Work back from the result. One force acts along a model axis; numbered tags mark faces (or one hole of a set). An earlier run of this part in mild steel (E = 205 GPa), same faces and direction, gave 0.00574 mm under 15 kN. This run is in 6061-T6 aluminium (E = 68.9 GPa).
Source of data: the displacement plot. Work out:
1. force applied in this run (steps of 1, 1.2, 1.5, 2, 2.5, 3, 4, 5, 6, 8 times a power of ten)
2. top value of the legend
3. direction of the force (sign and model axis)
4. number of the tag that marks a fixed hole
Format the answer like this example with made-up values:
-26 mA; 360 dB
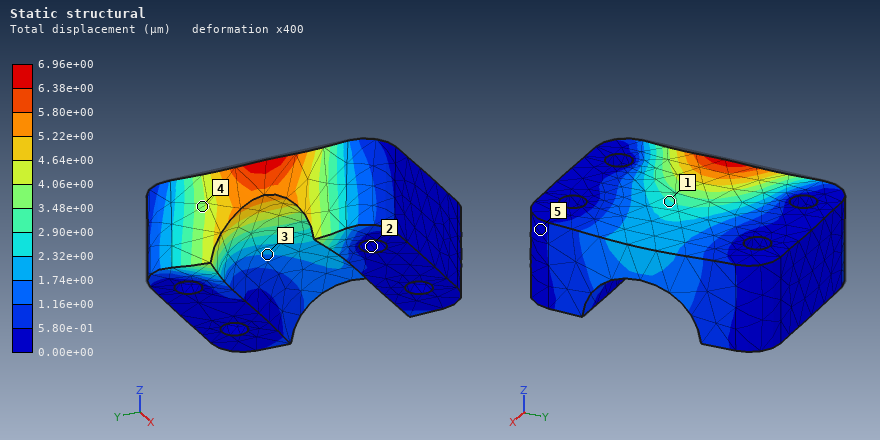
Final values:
6 kN; 6.96e+00 µm; +X; 2
